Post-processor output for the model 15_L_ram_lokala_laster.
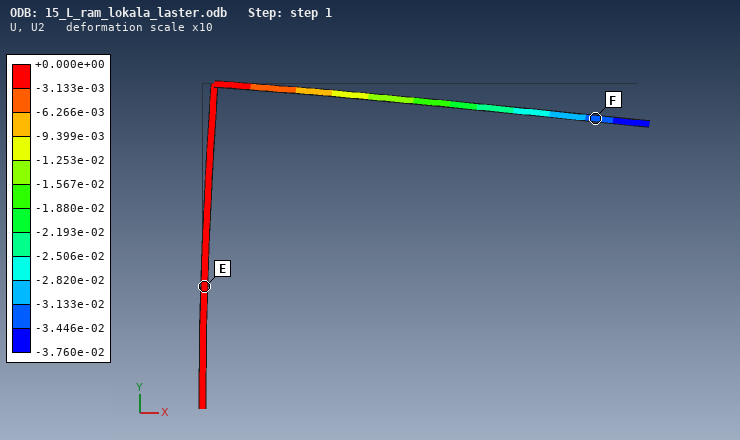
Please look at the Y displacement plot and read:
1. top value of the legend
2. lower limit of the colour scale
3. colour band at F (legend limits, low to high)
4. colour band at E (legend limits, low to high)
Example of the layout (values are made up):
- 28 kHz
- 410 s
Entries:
- +0.000e+00
- -3.760e-02
- -3.446e-02 to -3.133e-02
- -3.133e-03 to +0.000e+00
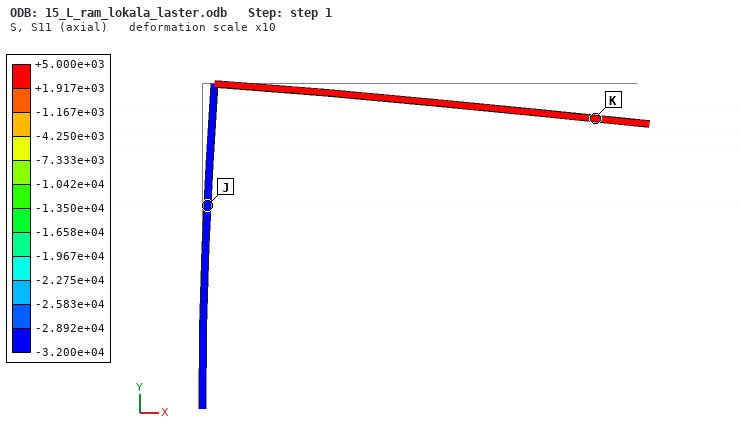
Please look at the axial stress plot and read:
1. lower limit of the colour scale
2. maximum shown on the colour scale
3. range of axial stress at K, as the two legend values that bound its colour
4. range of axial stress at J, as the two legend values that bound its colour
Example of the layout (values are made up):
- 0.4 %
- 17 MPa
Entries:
- -3.200e+04
- +5.000e+03
- +1.917e+03 to +5.000e+03
- -3.200e+04 to -2.892e+04
